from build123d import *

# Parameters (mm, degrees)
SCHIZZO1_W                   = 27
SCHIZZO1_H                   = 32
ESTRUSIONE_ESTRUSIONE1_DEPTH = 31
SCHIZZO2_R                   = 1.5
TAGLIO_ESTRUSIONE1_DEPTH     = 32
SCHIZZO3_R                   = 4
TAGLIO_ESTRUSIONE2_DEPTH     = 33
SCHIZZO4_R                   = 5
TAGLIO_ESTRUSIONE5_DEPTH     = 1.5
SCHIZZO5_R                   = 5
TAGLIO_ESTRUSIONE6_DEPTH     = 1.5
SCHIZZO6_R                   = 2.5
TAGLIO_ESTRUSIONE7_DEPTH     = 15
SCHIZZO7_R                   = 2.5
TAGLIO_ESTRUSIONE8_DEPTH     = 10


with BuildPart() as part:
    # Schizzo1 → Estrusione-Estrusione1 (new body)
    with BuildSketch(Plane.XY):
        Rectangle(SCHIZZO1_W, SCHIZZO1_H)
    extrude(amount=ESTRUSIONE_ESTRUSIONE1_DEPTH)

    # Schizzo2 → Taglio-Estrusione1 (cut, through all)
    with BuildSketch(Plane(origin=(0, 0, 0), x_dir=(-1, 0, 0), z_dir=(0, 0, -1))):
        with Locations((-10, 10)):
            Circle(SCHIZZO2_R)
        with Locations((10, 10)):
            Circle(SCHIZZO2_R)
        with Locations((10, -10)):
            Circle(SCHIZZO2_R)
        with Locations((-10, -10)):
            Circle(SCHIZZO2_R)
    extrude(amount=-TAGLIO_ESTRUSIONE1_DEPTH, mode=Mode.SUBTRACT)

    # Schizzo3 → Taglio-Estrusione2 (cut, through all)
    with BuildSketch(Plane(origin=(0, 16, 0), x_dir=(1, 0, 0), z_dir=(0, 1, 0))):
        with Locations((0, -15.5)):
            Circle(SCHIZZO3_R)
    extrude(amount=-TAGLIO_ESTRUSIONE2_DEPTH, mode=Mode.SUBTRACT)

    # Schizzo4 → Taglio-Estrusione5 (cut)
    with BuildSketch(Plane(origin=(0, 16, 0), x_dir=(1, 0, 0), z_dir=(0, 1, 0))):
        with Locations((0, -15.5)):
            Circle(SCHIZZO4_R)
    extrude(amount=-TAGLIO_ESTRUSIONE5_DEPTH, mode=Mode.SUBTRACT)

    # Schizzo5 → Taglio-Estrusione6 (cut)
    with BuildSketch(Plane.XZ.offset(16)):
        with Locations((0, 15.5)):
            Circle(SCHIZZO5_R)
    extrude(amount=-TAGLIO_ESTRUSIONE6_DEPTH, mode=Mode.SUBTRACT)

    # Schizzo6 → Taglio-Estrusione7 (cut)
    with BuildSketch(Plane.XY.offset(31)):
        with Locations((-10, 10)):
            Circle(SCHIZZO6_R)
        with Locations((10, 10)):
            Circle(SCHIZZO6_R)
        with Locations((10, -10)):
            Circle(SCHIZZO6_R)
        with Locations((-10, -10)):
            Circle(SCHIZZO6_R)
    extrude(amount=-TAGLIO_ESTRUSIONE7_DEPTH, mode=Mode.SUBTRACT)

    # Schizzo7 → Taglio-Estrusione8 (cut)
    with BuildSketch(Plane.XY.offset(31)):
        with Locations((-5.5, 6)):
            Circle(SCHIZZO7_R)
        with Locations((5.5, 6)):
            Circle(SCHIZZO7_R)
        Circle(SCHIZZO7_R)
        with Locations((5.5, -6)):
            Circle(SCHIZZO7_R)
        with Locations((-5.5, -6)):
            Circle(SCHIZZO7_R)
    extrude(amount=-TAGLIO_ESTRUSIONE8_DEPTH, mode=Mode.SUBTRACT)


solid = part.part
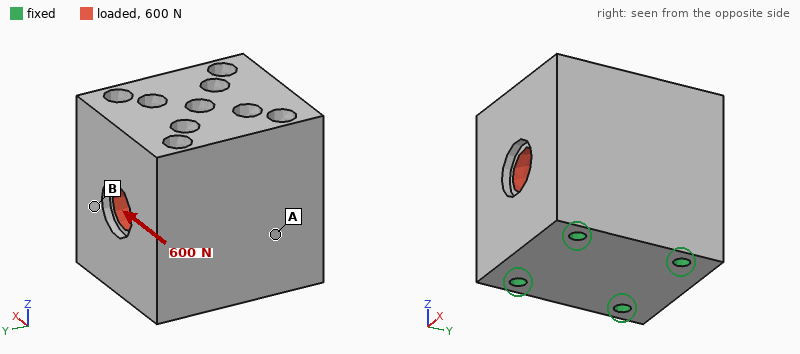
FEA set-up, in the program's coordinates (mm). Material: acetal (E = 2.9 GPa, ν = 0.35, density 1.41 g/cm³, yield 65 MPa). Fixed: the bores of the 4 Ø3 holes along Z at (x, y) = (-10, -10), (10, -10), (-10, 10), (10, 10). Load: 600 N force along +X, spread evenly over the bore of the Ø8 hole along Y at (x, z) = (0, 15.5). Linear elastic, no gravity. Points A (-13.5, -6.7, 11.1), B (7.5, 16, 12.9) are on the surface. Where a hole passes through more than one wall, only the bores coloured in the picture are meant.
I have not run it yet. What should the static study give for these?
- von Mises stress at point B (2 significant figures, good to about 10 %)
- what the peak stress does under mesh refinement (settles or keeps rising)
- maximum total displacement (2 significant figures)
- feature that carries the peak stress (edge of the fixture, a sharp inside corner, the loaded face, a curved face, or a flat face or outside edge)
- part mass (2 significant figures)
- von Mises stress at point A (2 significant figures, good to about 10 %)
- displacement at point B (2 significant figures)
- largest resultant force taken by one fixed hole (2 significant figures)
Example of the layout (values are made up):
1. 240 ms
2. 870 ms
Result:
1. 0.42 MPa
2. keeps rising
3. 9.0 µm
4. edge of the fixture
5. 32 g
6. 0.79 MPa
7. 2.1 µm
8. 160 N
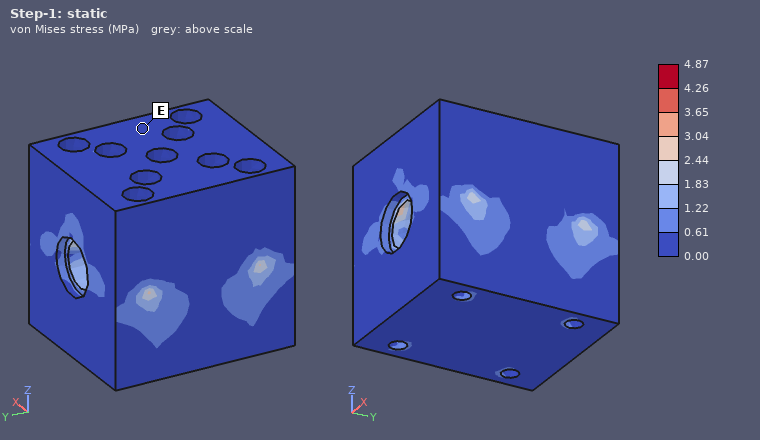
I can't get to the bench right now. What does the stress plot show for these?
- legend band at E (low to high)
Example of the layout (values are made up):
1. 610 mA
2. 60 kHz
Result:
1. 0.00 to 0.61 MPa
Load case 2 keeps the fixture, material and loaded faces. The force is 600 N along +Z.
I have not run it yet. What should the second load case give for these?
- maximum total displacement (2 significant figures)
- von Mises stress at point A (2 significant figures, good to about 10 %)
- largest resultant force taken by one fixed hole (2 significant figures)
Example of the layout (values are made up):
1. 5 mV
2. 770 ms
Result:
1. 8.1 µm
2. 0.64 MPa
3. 150 N
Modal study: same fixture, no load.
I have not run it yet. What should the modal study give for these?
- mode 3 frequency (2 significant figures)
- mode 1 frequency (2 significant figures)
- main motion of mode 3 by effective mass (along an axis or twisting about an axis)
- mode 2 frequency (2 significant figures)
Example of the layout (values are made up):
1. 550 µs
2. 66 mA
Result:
1. 9500 Hz
2. 7200 Hz
3. twisting about Z
4. 7500 Hz
